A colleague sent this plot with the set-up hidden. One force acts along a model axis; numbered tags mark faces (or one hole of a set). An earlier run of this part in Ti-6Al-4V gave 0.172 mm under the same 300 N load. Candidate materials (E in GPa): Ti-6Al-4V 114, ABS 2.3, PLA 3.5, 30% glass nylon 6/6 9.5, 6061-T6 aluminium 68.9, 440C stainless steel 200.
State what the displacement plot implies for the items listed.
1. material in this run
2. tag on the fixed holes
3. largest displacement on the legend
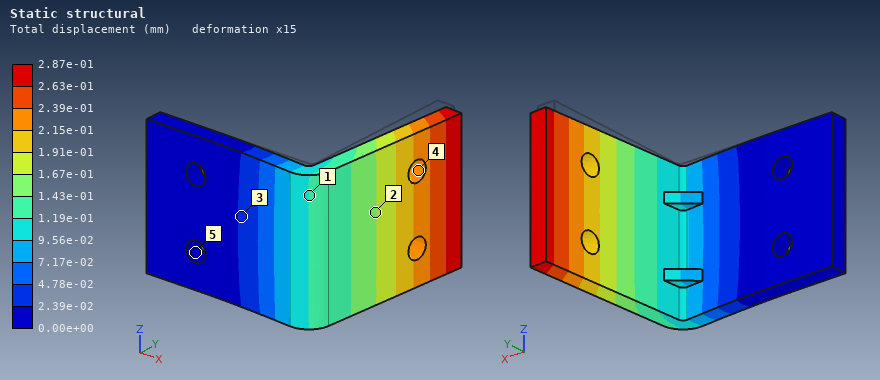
6061-T6 aluminium
5
2.87e-01 mm
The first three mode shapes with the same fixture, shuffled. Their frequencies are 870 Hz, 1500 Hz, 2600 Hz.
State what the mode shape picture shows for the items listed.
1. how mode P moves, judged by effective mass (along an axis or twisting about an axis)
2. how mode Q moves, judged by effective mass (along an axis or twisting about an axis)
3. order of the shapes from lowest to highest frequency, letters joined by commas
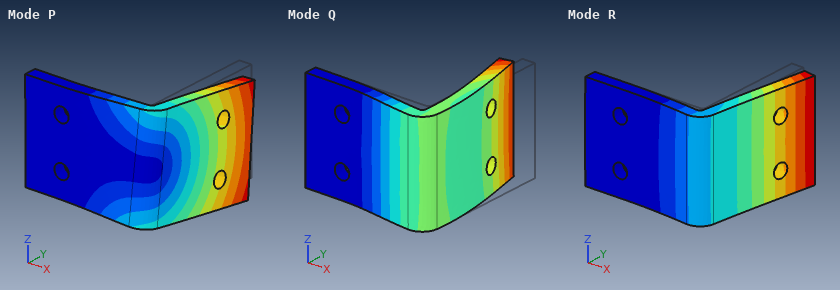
along Z
along Y
R, P, Q
